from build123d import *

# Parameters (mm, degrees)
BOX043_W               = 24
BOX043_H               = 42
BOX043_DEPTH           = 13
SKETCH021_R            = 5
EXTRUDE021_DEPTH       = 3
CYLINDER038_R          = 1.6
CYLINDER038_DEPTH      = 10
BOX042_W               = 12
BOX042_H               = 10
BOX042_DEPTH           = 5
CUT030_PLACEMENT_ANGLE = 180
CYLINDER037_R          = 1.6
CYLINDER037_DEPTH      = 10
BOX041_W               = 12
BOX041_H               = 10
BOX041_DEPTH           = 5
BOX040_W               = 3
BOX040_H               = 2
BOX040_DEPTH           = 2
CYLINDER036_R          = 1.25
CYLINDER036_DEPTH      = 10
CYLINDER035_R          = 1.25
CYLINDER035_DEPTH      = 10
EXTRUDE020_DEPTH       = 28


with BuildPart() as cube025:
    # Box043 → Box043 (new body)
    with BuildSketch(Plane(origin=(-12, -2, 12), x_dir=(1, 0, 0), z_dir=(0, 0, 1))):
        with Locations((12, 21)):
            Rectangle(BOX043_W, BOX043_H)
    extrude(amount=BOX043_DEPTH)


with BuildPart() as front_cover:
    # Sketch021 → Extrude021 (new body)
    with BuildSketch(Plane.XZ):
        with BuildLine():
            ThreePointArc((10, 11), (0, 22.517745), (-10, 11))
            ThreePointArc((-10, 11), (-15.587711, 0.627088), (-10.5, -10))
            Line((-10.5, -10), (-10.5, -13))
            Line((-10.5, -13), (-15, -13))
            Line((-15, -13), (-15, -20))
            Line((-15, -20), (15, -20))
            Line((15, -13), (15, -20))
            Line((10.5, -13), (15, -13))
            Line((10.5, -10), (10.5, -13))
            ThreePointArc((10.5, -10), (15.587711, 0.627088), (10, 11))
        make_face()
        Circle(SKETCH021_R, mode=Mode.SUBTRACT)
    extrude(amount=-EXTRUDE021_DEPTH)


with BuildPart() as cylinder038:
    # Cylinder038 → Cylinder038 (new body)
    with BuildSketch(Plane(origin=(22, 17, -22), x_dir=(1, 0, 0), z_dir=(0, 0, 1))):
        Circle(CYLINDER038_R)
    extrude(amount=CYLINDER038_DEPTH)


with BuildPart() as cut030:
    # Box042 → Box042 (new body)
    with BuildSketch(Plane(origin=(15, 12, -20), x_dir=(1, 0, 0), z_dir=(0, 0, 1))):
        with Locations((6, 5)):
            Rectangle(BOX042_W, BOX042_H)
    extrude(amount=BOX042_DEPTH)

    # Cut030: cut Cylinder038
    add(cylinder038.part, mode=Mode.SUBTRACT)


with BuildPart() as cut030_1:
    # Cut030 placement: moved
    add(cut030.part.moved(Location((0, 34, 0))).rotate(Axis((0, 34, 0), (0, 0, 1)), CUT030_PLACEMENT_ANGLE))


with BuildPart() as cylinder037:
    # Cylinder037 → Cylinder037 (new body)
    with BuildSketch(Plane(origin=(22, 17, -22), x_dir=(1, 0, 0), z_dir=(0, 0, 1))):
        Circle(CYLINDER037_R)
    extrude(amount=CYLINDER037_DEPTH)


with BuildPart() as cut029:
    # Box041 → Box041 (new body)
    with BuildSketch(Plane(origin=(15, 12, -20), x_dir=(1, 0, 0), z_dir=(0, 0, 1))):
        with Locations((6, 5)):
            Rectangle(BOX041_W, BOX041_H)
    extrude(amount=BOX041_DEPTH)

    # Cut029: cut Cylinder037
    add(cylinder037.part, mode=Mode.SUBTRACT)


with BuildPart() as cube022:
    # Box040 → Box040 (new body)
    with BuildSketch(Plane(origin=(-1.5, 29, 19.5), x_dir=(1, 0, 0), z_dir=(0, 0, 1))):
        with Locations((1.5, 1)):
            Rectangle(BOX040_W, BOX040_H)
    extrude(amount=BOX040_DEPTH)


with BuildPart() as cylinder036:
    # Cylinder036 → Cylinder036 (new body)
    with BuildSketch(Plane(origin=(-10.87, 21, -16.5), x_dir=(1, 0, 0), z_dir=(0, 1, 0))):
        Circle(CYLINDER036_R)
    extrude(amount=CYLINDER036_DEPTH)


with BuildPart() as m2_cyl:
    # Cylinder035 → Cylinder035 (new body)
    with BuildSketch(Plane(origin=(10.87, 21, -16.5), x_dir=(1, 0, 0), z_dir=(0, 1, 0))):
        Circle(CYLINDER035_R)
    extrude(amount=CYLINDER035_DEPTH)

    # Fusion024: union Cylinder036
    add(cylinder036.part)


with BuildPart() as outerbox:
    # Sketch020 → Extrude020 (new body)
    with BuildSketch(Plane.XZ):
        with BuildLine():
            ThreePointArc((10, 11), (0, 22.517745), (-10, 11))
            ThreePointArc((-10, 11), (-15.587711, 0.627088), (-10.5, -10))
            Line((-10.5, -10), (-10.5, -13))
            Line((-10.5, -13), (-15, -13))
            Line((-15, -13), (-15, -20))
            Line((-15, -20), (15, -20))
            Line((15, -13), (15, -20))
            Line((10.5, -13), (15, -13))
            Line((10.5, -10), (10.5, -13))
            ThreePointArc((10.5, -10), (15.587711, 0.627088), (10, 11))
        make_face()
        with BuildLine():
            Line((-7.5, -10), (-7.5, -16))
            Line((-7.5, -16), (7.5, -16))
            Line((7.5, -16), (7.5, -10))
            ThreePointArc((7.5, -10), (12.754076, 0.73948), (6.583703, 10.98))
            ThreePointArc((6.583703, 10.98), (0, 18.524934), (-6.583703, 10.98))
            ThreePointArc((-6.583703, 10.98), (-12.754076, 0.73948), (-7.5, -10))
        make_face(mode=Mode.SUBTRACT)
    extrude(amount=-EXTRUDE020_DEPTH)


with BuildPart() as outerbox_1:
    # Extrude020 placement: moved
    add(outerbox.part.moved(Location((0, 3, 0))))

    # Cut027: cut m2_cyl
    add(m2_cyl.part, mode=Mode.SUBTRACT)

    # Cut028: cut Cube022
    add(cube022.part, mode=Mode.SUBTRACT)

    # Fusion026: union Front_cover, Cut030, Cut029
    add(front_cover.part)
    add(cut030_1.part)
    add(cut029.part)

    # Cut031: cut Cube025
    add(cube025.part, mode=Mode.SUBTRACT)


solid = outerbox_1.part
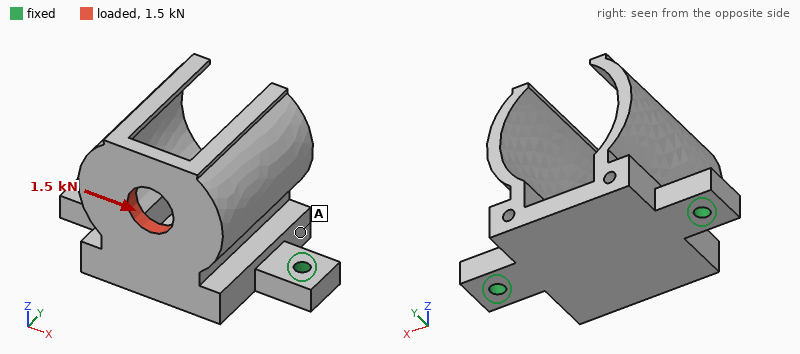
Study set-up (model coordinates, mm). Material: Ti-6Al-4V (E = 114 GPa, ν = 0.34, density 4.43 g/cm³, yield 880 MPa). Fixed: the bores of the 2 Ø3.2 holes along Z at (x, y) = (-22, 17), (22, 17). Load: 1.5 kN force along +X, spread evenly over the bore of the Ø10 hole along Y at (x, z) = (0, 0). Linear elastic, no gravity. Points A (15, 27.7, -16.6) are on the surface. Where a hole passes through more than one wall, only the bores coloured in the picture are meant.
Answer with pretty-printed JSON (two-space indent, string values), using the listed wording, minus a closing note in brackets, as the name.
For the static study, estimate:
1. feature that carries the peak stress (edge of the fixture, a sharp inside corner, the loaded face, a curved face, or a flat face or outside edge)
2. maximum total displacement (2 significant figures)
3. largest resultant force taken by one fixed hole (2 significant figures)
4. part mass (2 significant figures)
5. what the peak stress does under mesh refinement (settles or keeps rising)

{
  "feature that carries the peak stress": "edge of the fixture",
  "maximum total displacement": "0.10 mm",
  "largest resultant force taken by one fixed hole": "1.2 kN",
  "part mass": "54 g",
  "what the peak stress does under mesh refinement": "keeps rising"
}
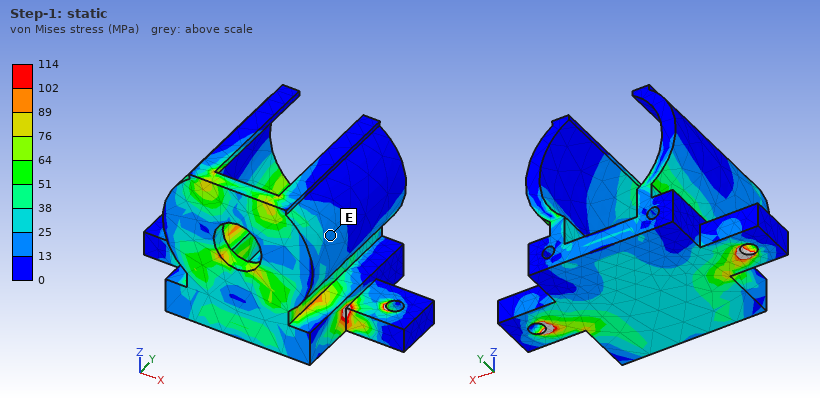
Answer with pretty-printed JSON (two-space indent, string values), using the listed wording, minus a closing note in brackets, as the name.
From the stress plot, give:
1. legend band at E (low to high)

{
  "legend band at E": "13 to 25 MPa"
}
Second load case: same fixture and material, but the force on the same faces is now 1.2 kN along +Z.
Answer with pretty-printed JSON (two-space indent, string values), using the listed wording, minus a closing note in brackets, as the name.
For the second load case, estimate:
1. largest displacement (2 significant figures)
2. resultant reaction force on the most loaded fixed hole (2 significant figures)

{
  "largest displacement": "0.22 mm",
  "resultant reaction force on the most loaded fixed hole": "600 N"
}
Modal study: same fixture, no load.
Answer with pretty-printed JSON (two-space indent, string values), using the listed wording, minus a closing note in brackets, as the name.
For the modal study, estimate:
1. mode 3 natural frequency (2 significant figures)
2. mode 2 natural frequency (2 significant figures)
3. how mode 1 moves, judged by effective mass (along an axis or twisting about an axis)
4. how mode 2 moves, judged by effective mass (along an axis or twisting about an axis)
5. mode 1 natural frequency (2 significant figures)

{
  "mode 3 natural frequency": "4400 Hz",
  "mode 2 natural frequency": "3900 Hz",
  "how mode 1 moves, judged by effective mass": "along Y",
  "how mode 2 moves, judged by effective mass": "along X",
  "mode 1 natural frequency": "2300 Hz"
}
